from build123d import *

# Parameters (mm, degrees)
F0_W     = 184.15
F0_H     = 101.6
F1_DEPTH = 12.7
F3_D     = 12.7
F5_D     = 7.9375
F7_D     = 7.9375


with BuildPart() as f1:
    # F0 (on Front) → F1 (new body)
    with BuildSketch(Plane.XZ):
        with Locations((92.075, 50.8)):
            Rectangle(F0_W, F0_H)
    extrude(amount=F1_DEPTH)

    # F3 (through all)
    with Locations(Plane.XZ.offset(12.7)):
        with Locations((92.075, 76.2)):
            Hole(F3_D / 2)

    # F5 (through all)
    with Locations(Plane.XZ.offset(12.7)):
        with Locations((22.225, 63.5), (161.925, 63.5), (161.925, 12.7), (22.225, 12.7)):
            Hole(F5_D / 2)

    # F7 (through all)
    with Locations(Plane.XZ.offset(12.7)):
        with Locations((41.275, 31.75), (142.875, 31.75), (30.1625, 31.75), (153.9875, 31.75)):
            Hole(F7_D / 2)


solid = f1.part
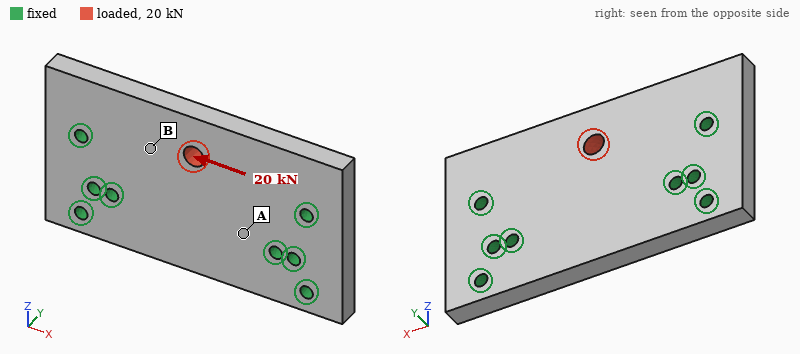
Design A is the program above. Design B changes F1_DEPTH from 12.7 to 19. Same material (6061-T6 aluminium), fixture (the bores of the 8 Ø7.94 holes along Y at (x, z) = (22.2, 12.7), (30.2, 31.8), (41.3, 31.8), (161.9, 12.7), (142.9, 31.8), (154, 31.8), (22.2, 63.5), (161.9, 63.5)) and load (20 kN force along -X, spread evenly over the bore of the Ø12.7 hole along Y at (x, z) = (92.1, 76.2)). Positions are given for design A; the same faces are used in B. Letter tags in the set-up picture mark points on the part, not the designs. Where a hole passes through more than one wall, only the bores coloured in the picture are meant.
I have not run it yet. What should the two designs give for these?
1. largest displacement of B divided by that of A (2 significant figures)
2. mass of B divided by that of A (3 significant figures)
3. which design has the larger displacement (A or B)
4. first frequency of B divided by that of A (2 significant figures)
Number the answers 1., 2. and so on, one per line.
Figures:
1. 0.67
2. 1.50
3. A
4. 1.4
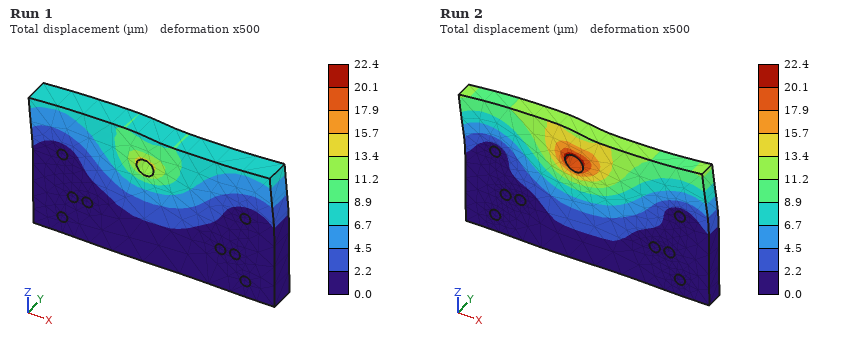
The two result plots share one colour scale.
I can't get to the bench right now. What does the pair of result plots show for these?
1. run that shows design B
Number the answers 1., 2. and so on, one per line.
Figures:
1. Run 1
